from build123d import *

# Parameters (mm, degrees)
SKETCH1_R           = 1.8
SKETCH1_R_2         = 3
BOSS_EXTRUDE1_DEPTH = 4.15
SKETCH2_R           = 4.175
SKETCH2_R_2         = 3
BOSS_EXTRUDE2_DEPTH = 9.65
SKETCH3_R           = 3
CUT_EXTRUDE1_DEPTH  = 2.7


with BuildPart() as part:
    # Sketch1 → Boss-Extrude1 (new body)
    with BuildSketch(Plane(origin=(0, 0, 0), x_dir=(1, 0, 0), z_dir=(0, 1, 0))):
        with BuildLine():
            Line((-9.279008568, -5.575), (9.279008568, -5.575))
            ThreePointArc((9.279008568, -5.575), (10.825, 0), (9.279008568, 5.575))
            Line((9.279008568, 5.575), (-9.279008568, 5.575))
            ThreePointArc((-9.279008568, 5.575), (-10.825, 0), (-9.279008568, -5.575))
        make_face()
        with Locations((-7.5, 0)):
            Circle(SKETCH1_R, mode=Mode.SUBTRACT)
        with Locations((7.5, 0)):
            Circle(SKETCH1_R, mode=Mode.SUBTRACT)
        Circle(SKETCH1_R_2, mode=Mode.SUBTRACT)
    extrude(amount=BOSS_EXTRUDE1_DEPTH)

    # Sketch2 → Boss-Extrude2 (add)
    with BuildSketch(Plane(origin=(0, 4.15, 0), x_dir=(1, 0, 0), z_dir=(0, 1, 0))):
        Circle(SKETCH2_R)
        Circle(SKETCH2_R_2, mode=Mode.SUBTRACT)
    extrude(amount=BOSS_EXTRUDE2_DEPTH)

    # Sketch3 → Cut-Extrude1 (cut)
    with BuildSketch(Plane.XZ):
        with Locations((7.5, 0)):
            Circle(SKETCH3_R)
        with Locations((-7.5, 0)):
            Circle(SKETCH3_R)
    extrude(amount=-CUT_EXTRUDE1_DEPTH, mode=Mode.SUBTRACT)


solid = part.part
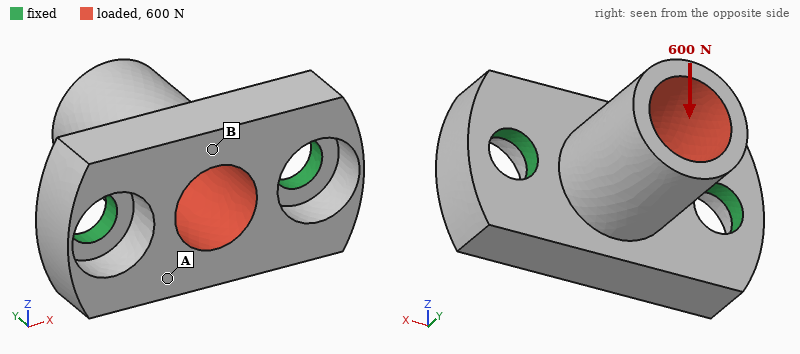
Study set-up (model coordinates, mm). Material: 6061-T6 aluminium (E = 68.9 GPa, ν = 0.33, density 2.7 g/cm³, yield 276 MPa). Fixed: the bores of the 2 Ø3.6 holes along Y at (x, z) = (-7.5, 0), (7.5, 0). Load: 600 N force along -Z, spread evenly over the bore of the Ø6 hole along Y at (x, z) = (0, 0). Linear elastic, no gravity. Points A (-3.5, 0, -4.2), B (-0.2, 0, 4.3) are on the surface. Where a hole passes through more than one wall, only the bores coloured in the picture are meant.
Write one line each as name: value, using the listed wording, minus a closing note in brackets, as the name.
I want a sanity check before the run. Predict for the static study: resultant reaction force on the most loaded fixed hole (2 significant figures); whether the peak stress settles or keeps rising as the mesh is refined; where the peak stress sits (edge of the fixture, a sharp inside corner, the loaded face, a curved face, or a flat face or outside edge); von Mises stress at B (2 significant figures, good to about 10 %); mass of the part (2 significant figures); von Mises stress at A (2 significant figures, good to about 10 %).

resultant reaction force on the most loaded fixed hole: 300 N
whether the peak stress settles or keeps rising as the mesh is refined: keeps rising
where the peak stress sits: edge of the fixture
von Mises stress at B: 50 MPa
mass of the part: 2.5 g
von Mises stress at A: 24 MPa
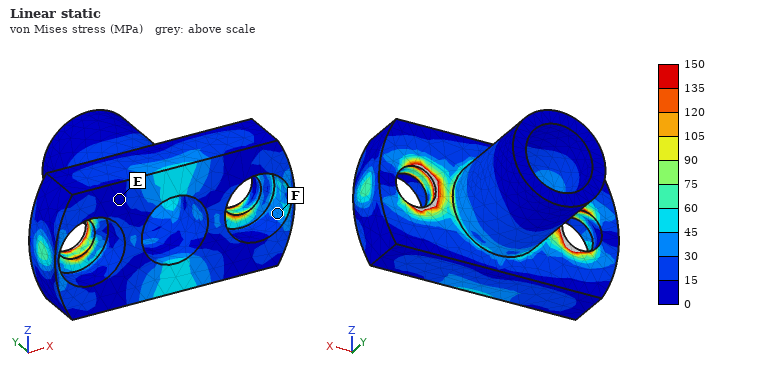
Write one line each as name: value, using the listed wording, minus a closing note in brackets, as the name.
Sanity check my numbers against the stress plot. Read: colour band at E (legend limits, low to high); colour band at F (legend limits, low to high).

colour band at E: 0 to 15 MPa
colour band at F: 30 to 45 MPa
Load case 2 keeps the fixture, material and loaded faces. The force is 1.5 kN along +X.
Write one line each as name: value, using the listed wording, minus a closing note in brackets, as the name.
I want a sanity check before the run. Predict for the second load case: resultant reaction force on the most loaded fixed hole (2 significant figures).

resultant reaction force on the most loaded fixed hole: 880 N
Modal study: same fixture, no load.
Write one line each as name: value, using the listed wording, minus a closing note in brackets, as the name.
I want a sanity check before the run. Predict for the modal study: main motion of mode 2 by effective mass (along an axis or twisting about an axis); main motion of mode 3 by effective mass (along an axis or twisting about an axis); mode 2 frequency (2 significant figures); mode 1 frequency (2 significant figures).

main motion of mode 2 by effective mass: along X
main motion of mode 3 by effective mass: along Y
mode 2 frequency: 33 kHz
mode 1 frequency: 18 kHz
